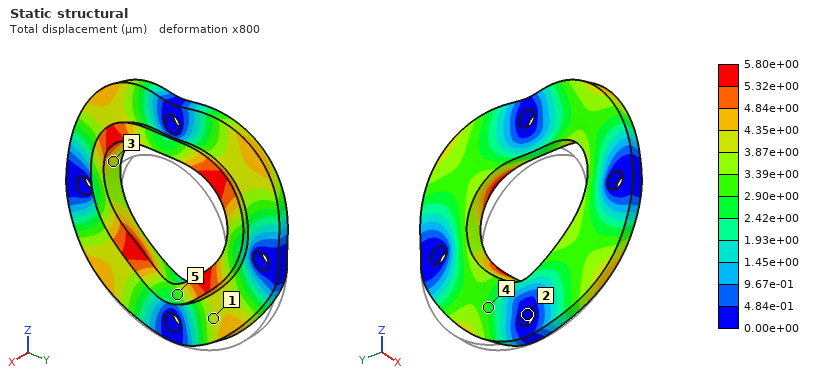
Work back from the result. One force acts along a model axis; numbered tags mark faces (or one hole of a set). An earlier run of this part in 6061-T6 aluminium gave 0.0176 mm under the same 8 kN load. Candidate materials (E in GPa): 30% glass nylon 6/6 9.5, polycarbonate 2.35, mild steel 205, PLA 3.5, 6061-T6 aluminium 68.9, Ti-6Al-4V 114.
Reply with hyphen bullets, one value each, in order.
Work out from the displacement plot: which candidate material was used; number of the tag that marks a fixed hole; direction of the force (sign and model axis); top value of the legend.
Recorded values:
- mild steel
- 2
- +Z
- 5.80e+00 µm
